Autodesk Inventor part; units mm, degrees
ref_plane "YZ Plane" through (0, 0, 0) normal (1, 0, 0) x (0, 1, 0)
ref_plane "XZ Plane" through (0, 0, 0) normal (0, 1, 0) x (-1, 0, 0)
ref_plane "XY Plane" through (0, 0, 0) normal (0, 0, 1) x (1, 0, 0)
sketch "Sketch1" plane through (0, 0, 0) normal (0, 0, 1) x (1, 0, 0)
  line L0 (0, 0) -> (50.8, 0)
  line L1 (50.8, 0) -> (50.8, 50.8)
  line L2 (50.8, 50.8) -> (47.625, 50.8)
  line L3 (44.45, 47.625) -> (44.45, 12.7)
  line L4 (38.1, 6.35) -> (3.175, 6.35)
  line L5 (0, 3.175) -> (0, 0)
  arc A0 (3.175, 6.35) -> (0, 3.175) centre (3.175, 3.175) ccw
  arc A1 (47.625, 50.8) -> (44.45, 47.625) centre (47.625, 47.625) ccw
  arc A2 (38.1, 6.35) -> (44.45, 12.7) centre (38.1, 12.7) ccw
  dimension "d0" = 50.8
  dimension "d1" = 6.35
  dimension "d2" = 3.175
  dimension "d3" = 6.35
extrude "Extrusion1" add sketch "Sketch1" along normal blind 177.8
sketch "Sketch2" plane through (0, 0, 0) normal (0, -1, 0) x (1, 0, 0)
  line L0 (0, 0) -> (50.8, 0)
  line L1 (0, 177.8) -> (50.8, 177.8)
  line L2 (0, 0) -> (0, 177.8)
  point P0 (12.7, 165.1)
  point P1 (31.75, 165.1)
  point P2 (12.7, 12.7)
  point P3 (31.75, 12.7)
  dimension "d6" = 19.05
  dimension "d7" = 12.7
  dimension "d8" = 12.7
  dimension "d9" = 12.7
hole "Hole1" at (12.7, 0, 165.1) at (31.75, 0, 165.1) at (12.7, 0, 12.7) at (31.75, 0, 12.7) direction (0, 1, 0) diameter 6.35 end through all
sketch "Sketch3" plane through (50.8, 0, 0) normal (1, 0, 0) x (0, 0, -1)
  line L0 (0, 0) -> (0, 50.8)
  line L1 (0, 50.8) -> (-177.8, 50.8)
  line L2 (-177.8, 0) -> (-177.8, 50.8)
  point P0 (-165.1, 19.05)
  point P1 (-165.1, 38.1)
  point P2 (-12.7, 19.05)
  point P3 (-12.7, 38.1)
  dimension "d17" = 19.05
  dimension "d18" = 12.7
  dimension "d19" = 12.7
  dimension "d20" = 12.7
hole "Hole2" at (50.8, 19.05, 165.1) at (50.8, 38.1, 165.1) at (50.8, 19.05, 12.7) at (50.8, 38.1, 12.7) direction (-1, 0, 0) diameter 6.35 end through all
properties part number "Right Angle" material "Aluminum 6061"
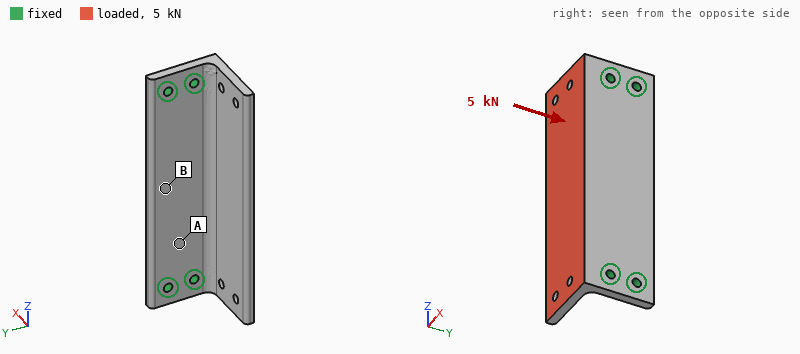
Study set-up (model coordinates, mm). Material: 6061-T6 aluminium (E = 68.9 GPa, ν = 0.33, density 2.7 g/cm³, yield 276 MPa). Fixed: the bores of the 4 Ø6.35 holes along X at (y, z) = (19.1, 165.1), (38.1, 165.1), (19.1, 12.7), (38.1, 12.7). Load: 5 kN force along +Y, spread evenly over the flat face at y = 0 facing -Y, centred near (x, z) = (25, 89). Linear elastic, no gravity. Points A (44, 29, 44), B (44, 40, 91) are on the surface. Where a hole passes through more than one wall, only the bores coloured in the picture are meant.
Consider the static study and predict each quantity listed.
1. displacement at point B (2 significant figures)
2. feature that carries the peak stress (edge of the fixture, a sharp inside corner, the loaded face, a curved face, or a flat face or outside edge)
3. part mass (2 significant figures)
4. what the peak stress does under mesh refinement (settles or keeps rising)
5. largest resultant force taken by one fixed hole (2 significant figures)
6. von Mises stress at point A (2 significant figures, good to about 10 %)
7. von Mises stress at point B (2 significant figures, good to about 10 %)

0.22 mm
edge of the fixture
290 g
keeps rising
2.5 kN
58 MPa
21 MPa
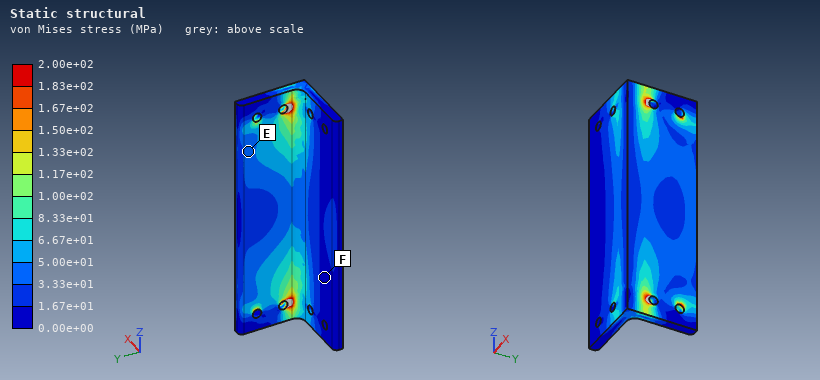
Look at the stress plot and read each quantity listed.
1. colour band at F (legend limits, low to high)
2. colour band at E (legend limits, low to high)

0.00e+00 to 1.67e+01 MPa
3.33e+01 to 5.00e+01 MPa
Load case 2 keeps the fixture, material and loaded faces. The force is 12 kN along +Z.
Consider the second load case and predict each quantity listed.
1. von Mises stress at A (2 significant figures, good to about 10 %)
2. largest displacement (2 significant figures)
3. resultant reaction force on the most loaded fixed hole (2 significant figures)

15 MPa
66 µm
4.9 kN
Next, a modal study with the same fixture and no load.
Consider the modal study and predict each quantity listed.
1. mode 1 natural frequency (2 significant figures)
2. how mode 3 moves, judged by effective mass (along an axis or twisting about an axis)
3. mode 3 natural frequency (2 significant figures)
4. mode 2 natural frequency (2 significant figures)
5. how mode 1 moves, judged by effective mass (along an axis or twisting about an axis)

1300 Hz
along X
2500 Hz
2100 Hz
along Y
